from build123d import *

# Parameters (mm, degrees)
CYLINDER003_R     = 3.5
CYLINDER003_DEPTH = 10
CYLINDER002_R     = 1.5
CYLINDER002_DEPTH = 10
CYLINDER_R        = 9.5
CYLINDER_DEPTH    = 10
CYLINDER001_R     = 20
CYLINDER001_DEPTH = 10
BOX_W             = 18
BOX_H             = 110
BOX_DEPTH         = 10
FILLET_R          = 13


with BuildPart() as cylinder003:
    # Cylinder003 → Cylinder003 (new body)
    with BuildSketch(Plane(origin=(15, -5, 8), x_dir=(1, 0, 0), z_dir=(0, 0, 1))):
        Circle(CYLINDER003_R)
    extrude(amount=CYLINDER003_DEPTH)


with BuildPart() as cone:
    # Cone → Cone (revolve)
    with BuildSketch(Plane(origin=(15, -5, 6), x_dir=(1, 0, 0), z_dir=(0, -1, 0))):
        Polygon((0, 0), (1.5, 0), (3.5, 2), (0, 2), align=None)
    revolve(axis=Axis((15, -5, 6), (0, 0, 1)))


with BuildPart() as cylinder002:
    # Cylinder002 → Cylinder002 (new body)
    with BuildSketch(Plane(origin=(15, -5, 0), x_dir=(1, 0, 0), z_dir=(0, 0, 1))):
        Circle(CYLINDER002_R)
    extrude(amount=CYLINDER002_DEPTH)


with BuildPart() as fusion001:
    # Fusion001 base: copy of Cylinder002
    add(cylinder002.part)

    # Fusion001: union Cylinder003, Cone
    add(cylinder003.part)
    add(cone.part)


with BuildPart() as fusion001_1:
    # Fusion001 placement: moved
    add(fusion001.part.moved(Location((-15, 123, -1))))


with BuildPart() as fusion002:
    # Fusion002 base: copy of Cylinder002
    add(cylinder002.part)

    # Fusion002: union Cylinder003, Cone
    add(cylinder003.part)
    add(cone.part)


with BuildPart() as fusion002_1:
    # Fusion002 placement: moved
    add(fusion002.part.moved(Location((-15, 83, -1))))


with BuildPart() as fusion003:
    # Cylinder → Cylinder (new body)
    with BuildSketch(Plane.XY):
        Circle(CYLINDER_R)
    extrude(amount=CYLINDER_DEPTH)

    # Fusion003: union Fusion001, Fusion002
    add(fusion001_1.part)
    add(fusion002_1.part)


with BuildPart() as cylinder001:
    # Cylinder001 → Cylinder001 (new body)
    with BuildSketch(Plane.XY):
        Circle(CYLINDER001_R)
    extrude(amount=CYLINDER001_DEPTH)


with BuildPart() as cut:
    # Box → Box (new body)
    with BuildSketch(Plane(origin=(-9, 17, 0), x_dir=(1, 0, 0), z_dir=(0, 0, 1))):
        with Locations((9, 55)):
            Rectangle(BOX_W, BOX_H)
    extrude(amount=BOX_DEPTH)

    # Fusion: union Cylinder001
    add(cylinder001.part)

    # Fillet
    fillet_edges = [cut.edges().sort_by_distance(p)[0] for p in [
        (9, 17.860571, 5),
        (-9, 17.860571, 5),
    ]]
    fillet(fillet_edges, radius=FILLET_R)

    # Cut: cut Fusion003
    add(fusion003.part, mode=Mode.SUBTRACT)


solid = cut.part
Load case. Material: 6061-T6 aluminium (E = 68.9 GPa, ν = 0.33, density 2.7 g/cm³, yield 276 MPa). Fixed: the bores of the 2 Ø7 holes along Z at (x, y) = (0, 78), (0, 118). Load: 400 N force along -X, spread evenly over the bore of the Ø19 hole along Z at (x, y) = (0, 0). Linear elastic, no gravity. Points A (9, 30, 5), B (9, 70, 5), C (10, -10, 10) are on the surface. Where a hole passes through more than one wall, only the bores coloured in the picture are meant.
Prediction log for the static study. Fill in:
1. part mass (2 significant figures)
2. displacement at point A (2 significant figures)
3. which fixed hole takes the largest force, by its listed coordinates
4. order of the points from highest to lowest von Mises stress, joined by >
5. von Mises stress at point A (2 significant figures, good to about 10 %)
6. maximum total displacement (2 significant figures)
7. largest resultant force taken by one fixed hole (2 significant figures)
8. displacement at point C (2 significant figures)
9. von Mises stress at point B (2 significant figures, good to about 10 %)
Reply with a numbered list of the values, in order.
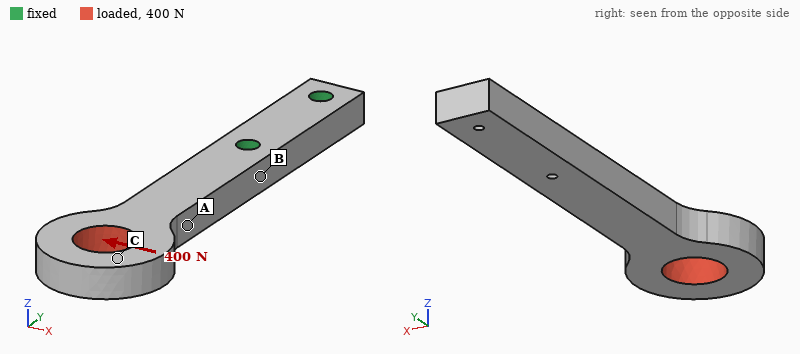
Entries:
1. 78 g
2. 0.13 mm
3. (0, 78)
4. B > A > C
5. 22 MPa
6. 0.34 mm
7. 850 N
8. 0.30 mm
9. 52 MPa
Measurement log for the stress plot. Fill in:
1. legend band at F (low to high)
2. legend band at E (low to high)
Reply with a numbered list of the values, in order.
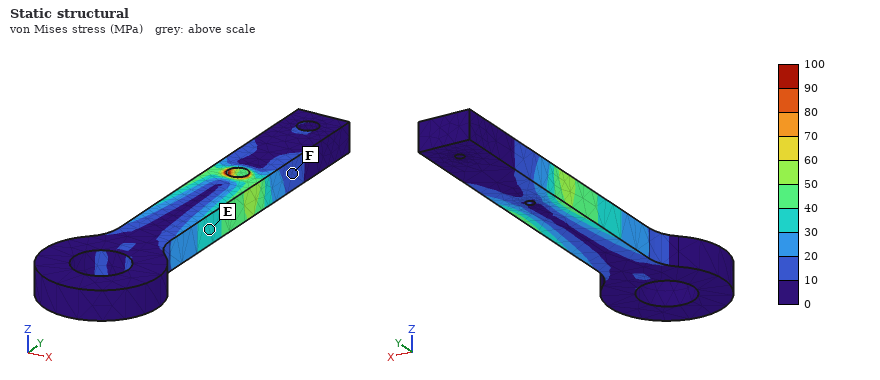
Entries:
1. 10 to 20 MPa
2. 30 to 40 MPa
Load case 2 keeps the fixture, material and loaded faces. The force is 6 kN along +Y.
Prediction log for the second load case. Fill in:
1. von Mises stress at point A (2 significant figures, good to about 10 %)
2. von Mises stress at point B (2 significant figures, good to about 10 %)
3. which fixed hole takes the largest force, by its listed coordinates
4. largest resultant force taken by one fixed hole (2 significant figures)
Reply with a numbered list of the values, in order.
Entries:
1. 33 MPa
2. 27 MPa
3. (0, 78)
4. 4.8 kN
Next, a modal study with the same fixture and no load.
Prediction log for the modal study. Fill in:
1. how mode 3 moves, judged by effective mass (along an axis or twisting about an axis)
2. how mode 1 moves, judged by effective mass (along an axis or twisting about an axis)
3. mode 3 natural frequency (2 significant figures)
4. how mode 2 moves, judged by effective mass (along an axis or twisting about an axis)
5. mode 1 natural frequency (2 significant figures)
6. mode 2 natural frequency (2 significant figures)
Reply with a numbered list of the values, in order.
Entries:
1. twisting about Y
2. along Z
3. 3000 Hz
4. along X
5. 690 Hz
6. 1100 Hz
